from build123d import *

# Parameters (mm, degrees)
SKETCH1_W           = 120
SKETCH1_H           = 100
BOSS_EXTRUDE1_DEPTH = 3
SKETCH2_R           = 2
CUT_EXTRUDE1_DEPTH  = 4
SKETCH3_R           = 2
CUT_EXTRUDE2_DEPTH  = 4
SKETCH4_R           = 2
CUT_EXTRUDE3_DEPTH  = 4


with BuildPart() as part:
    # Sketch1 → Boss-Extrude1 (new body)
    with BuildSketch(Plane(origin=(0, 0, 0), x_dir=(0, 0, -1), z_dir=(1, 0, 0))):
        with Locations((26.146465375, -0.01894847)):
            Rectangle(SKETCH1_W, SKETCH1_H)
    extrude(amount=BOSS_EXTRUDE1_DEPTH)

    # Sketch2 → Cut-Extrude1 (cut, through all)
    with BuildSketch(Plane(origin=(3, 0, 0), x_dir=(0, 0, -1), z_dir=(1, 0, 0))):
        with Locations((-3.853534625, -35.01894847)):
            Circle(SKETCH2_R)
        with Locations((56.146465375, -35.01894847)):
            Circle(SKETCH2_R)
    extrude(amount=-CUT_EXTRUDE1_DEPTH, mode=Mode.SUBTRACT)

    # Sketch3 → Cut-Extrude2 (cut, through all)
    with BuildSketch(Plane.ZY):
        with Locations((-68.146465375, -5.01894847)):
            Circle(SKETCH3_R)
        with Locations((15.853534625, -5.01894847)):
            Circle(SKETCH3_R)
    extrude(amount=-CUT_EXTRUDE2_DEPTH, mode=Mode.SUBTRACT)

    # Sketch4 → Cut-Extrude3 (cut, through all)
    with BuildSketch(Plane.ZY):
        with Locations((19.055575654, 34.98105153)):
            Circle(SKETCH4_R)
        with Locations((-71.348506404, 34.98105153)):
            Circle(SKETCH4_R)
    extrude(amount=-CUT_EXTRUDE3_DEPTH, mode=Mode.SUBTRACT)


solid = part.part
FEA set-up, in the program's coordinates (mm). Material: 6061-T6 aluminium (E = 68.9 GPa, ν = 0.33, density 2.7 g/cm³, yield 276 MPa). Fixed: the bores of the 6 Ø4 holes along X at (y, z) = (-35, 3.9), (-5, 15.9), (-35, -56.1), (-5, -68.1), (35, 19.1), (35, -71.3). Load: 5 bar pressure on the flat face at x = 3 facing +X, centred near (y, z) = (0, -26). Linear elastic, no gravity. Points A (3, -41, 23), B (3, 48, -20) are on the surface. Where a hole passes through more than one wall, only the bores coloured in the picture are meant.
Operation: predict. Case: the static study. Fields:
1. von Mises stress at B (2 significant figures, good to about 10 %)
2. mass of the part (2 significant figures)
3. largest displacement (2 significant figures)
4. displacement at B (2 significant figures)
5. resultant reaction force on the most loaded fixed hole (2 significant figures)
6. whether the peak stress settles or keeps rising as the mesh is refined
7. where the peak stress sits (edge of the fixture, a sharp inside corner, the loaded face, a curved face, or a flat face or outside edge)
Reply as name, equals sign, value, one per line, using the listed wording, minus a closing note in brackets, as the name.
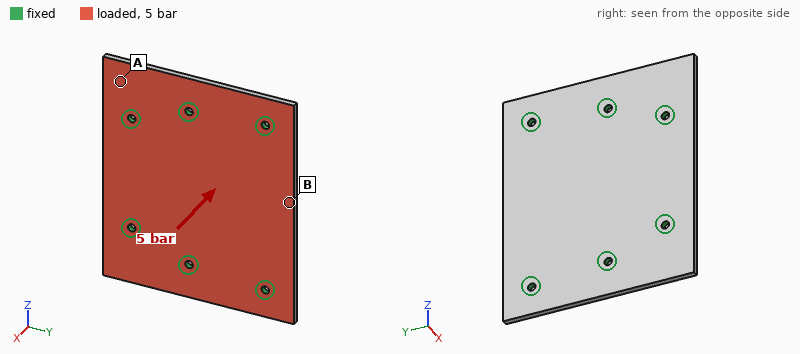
von Mises stress at B = 110 MPa
mass of the part = 97 g
largest displacement = 0.67 mm
displacement at B = 0.63 mm
resultant reaction force on the most loaded fixed hole = 1.0 kN
whether the peak stress settles or keeps rising as the mesh is refined = keeps rising
where the peak stress sits = edge of the fixture
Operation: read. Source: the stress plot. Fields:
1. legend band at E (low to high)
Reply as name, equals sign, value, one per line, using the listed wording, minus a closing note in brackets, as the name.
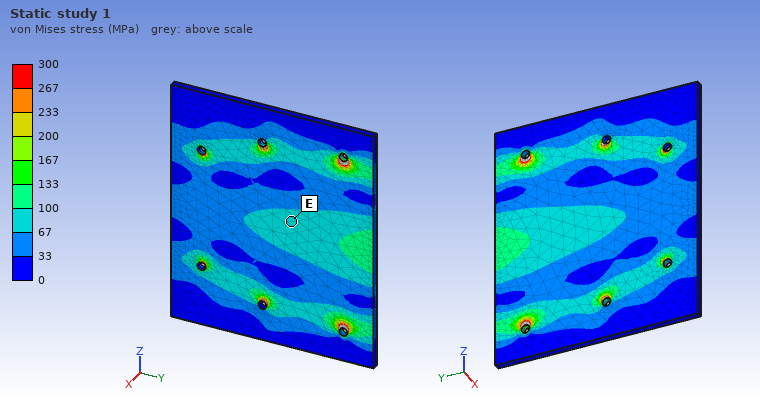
legend band at E = 67 to 100 MPa
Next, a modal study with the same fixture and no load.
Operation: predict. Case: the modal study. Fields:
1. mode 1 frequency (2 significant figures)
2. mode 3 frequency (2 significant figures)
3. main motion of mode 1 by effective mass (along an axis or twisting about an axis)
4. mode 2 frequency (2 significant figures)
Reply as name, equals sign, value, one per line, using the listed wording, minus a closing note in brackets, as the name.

mode 1 frequency = 2000 Hz
mode 3 frequency = 3400 Hz
main motion of mode 1 by effective mass = along X
mode 2 frequency = 3100 Hz
